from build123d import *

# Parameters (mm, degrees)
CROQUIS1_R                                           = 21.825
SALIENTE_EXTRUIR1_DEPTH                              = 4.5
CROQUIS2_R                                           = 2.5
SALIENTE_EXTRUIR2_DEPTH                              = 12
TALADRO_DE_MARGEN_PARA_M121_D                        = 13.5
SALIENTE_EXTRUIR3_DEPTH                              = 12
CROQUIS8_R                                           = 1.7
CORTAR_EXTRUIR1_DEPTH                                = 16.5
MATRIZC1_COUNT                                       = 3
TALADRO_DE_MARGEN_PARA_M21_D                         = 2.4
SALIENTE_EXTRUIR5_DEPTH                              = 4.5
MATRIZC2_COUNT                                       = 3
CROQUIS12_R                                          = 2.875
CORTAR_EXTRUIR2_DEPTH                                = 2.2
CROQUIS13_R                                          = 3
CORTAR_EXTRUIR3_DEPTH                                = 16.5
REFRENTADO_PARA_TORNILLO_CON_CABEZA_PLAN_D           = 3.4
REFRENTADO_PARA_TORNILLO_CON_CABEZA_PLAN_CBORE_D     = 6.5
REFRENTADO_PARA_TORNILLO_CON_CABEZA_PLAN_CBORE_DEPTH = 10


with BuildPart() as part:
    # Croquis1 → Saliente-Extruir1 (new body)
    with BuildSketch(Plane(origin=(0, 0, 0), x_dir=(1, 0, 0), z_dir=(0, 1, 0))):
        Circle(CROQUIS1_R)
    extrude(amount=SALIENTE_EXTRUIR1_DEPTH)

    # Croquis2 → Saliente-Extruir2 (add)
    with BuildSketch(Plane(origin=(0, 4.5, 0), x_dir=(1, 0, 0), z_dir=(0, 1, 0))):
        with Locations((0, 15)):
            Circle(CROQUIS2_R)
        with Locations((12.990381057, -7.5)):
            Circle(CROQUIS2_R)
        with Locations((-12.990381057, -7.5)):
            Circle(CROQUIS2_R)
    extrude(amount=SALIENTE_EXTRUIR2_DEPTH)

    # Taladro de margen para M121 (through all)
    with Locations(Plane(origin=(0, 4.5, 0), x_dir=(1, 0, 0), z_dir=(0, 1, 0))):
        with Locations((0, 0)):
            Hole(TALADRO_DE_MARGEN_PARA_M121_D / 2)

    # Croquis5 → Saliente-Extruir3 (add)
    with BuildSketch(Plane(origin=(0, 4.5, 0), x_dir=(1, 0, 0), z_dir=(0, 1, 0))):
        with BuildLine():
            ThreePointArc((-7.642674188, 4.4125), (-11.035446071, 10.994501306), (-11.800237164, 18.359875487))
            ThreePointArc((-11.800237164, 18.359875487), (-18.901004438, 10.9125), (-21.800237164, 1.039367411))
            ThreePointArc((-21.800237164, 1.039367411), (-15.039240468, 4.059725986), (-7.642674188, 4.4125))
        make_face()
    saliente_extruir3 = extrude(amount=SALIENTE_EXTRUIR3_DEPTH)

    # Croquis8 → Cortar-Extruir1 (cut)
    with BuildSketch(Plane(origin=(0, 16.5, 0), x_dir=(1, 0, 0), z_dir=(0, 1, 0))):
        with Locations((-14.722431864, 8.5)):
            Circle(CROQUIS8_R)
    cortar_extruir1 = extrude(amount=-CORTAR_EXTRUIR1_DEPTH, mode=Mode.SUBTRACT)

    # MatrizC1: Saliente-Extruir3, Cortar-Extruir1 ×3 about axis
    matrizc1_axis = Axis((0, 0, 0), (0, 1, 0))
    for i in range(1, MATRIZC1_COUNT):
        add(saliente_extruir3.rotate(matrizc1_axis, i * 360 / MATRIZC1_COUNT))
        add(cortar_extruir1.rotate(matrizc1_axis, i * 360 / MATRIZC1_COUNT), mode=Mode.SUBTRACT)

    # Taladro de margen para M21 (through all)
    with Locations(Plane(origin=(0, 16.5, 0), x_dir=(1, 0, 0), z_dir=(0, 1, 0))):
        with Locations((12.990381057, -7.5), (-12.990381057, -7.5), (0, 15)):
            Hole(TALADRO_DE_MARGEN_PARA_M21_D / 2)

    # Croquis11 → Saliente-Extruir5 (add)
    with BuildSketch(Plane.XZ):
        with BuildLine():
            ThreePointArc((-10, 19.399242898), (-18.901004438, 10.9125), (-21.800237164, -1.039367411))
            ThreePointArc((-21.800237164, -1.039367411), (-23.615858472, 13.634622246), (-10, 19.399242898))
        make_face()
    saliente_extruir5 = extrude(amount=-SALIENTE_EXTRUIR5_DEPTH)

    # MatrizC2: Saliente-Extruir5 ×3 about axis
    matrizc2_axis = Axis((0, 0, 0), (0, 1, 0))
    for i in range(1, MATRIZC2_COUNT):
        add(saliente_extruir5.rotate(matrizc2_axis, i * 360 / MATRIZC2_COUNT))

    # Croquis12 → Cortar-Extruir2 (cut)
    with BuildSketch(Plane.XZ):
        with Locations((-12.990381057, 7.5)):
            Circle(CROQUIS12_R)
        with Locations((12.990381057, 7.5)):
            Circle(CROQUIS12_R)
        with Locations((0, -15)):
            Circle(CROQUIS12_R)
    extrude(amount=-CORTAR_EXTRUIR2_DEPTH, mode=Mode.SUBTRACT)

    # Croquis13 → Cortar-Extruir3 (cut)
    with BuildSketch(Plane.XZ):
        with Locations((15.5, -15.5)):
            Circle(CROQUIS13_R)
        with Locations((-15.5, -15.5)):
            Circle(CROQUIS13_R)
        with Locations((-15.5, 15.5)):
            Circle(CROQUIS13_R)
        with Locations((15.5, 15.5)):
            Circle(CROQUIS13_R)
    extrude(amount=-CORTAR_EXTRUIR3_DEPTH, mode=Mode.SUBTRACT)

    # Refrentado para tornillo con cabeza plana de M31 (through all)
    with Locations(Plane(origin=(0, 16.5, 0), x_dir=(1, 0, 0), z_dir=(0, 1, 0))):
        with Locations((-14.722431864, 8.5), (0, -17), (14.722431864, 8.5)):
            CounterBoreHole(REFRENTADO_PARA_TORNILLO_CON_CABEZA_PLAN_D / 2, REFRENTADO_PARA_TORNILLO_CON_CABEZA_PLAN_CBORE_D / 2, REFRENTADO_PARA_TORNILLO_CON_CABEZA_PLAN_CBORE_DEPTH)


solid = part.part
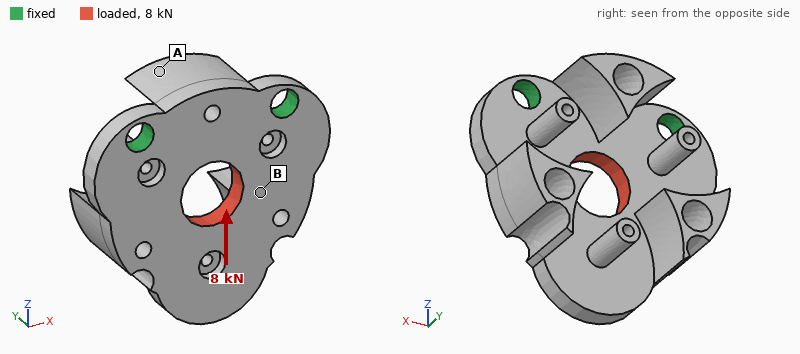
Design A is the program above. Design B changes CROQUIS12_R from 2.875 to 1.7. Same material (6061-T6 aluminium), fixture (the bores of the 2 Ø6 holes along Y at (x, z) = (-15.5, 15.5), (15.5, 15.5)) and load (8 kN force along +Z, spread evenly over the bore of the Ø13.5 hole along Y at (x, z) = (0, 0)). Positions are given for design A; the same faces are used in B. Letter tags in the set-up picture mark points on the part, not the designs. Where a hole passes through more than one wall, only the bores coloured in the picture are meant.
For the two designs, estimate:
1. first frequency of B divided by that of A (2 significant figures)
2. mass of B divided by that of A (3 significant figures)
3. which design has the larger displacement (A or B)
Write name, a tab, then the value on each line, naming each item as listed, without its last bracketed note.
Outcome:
first frequency of B divided by that of A	1.0
mass of B divided by that of A	1.01
which design has the larger displacement	A
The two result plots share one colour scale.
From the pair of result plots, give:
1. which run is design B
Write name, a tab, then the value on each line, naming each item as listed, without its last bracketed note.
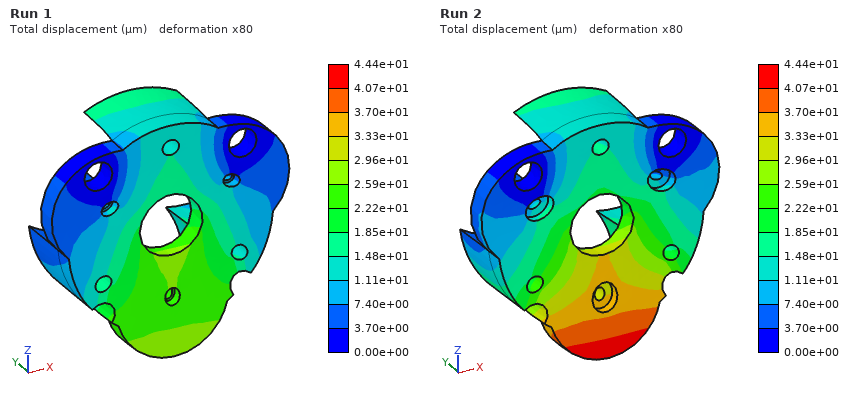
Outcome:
which run is design B	Run 1
